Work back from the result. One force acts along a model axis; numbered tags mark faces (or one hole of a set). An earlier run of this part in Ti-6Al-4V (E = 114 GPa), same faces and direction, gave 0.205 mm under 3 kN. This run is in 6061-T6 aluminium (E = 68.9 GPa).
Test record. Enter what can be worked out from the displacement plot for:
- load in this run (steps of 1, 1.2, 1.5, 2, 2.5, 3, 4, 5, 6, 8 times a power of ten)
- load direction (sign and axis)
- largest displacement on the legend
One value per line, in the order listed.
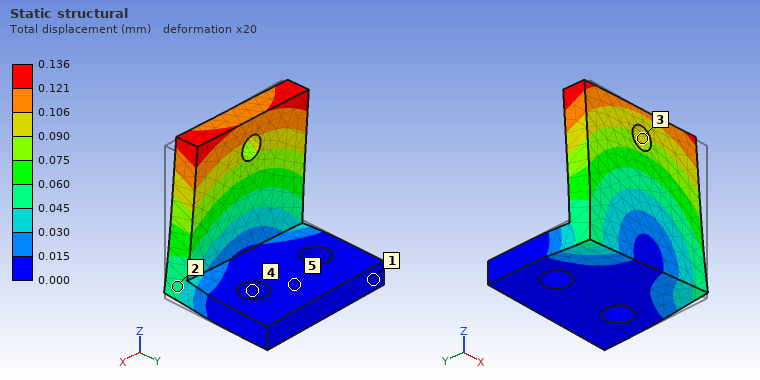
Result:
1.2 kN
-X
0.136 mm
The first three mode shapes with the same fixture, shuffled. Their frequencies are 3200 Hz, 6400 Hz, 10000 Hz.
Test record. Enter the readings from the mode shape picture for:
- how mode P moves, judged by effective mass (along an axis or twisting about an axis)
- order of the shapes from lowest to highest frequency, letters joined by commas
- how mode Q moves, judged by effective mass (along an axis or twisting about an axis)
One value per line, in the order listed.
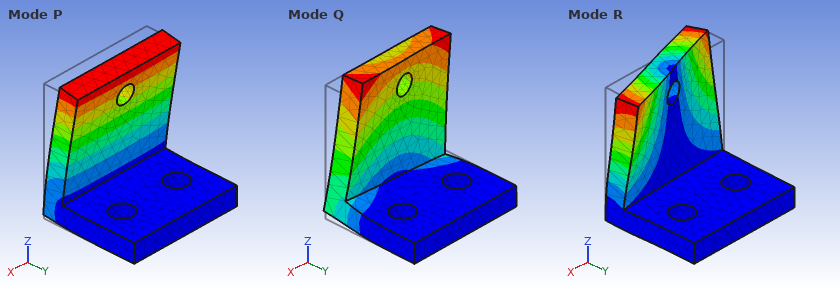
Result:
along Y
P, Q, R
along X
